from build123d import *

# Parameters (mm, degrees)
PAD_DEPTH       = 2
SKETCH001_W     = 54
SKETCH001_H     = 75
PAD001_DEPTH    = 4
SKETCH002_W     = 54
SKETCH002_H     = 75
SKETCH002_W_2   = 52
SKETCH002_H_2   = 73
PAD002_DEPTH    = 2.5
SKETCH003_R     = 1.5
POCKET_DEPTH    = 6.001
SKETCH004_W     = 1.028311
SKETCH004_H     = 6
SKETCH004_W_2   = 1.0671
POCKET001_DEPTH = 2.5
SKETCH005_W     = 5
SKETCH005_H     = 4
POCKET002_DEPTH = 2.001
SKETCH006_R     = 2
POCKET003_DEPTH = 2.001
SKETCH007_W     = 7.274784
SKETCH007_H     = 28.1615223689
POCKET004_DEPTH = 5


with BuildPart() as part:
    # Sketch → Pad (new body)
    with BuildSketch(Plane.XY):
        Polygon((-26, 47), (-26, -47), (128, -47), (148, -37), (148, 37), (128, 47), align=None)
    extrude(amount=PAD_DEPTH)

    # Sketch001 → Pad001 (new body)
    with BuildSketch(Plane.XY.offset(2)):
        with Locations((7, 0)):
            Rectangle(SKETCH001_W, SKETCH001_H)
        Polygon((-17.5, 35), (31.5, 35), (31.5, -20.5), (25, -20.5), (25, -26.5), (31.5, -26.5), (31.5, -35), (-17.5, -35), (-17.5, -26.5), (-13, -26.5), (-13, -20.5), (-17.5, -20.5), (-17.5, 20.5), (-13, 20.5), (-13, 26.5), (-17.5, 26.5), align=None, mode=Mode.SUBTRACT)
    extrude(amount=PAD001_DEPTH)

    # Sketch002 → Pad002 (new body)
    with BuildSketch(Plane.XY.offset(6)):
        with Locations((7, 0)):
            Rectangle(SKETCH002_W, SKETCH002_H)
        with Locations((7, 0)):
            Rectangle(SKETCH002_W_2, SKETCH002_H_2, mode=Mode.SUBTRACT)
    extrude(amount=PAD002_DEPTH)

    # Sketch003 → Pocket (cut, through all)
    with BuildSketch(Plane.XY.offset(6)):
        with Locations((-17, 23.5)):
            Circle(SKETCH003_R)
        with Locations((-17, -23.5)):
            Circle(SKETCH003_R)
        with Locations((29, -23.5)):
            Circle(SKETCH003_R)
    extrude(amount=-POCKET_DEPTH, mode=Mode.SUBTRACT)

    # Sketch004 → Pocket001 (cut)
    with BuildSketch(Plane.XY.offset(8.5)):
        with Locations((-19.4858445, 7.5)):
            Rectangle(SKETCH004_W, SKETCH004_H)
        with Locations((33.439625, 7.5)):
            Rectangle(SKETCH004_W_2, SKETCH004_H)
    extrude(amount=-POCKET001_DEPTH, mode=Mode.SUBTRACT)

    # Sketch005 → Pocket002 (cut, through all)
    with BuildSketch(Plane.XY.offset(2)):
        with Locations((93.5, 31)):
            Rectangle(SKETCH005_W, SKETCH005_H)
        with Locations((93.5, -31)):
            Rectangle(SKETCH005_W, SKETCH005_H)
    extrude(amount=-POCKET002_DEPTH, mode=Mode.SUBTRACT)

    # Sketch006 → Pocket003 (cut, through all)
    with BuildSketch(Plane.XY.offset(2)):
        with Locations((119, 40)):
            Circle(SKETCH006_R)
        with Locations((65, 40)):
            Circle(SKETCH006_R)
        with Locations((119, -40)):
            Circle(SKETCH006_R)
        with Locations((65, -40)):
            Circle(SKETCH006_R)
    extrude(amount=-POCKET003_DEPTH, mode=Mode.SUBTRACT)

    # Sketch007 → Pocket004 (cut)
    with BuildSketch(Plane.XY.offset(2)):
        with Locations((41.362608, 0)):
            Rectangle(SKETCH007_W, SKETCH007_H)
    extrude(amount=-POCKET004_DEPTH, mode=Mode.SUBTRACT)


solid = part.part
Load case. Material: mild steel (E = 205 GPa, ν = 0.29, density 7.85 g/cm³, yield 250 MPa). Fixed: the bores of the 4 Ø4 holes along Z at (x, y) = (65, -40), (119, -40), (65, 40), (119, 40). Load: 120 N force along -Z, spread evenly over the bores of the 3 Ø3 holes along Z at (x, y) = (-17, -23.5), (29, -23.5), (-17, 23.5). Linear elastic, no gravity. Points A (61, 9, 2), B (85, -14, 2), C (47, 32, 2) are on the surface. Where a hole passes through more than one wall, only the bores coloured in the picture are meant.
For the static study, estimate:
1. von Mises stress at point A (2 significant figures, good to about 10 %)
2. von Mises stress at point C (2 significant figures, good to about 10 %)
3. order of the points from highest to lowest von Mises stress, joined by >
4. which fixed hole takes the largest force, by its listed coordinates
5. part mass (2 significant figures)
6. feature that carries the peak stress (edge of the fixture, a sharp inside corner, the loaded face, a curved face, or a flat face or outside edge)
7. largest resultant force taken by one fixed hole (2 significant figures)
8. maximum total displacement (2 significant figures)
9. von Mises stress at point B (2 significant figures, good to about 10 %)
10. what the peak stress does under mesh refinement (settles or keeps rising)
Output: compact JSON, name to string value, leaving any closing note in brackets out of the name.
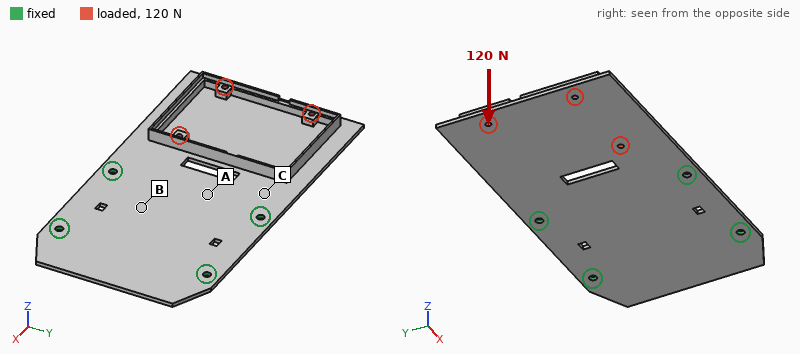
{"von Mises stress at point A": "60 MPa", "von Mises stress at point C": "110 MPa", "order of the points from highest to lowest von Mises stress, joined by >": "C > A > B", "which fixed hole takes the largest force, by its listed coordinates": "(65, -40)", "part mass": "280 g", "feature that carries the peak stress": "edge of the fixture", "largest resultant force taken by one fixed hole": "100 N", "maximum total displacement": "1.7 mm", "von Mises stress at point B": "24 MPa", "what the peak stress does under mesh refinement": "keeps rising"}
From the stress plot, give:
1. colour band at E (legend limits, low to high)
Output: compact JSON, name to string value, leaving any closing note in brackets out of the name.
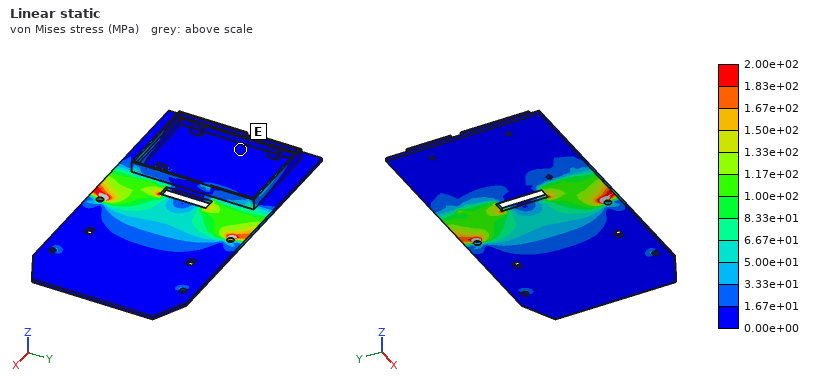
{"colour band at E": "0.00e+00 to 1.67e+01 MPa"}
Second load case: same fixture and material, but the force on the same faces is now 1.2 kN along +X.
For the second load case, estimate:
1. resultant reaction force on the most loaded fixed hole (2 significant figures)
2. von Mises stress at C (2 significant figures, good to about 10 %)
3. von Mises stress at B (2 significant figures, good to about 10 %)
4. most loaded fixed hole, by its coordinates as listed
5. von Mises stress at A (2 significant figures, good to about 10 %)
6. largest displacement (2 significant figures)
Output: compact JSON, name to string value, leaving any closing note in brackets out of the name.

{"resultant reaction force on the most loaded fixed hole": "570 N", "von Mises stress at C": "49 MPa", "von Mises stress at B": "9.7 MPa", "most loaded fixed hole, by its coordinates as listed": "(65, -40)", "von Mises stress at A": "22 MPa", "largest displacement": "0.65 mm"}
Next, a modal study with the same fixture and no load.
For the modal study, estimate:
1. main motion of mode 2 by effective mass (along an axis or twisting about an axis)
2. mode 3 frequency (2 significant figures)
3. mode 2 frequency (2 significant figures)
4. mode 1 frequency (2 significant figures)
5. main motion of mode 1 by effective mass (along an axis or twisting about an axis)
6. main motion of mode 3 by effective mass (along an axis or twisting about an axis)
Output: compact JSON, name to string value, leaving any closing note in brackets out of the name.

{"main motion of mode 2 by effective mass": "twisting about X", "mode 3 frequency": "1200 Hz", "mode 2 frequency": "500 Hz", "mode 1 frequency": "160 Hz", "main motion of mode 1 by effective mass": "along Z", "main motion of mode 3 by effective mass": "along Z"}
